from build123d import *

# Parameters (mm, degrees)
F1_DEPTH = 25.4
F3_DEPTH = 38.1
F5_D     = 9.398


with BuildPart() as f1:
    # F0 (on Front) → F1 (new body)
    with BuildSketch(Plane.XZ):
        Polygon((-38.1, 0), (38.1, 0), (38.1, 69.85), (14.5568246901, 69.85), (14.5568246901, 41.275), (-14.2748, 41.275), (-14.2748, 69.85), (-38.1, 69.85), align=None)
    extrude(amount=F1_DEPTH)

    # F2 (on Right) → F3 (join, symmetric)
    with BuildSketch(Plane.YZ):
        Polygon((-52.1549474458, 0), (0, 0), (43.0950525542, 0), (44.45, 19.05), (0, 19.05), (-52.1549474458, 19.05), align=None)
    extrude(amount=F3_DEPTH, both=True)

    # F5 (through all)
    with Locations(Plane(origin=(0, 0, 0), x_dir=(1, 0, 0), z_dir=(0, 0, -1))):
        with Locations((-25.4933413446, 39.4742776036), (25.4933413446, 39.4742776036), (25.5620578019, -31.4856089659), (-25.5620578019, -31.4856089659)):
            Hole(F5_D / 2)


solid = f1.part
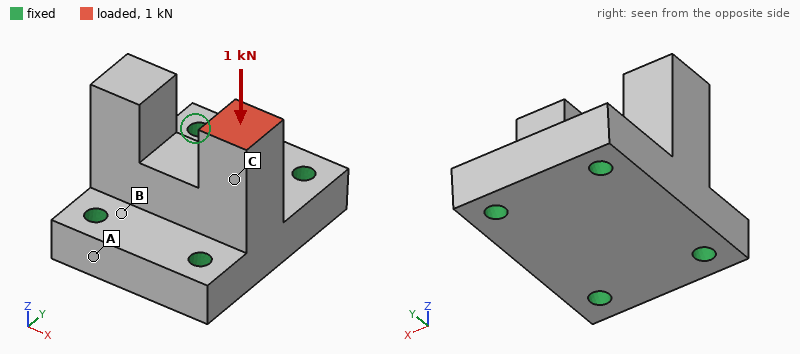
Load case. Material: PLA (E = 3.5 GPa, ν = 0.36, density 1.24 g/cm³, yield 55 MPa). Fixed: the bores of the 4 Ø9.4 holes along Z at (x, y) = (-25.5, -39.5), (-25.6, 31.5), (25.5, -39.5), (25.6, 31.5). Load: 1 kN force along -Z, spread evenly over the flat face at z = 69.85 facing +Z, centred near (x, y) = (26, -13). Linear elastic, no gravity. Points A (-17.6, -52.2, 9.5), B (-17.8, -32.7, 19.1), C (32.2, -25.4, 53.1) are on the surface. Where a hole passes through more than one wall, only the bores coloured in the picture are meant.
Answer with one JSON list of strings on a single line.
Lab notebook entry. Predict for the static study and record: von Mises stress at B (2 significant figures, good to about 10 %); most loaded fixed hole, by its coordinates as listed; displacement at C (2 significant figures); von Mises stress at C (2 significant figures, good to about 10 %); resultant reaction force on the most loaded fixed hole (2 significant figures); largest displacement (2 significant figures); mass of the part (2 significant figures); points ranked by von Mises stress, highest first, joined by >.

["0.91 MPa", "(25.5, -39.5)", "57 µm", "1.7 MPa", "640 N", "84 µm", "260 g", "C > B > A"]
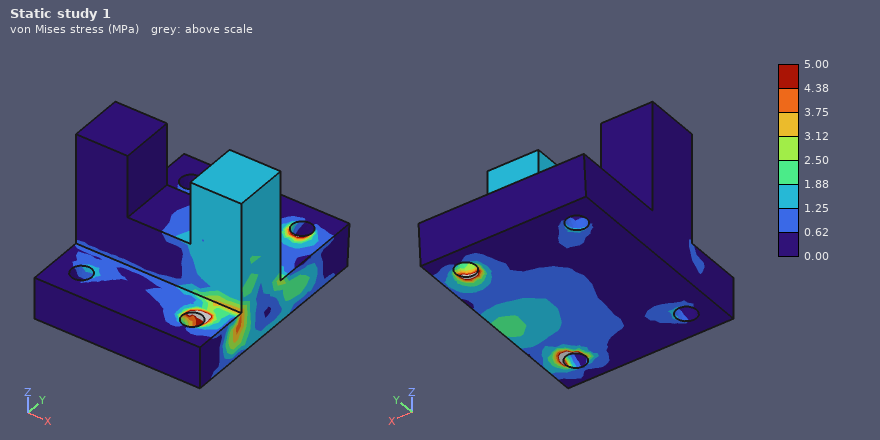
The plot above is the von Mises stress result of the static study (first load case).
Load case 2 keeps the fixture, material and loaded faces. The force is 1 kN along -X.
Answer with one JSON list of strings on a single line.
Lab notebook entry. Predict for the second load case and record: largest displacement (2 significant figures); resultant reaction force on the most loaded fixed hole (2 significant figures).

["0.42 mm", "860 N"]
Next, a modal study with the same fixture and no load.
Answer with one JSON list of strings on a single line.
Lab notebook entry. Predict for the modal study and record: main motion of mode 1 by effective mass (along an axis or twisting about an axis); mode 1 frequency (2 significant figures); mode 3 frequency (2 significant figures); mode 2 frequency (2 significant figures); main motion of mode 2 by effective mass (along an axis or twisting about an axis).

["along Y", "1800 Hz", "2200 Hz", "2000 Hz", "along X"]
